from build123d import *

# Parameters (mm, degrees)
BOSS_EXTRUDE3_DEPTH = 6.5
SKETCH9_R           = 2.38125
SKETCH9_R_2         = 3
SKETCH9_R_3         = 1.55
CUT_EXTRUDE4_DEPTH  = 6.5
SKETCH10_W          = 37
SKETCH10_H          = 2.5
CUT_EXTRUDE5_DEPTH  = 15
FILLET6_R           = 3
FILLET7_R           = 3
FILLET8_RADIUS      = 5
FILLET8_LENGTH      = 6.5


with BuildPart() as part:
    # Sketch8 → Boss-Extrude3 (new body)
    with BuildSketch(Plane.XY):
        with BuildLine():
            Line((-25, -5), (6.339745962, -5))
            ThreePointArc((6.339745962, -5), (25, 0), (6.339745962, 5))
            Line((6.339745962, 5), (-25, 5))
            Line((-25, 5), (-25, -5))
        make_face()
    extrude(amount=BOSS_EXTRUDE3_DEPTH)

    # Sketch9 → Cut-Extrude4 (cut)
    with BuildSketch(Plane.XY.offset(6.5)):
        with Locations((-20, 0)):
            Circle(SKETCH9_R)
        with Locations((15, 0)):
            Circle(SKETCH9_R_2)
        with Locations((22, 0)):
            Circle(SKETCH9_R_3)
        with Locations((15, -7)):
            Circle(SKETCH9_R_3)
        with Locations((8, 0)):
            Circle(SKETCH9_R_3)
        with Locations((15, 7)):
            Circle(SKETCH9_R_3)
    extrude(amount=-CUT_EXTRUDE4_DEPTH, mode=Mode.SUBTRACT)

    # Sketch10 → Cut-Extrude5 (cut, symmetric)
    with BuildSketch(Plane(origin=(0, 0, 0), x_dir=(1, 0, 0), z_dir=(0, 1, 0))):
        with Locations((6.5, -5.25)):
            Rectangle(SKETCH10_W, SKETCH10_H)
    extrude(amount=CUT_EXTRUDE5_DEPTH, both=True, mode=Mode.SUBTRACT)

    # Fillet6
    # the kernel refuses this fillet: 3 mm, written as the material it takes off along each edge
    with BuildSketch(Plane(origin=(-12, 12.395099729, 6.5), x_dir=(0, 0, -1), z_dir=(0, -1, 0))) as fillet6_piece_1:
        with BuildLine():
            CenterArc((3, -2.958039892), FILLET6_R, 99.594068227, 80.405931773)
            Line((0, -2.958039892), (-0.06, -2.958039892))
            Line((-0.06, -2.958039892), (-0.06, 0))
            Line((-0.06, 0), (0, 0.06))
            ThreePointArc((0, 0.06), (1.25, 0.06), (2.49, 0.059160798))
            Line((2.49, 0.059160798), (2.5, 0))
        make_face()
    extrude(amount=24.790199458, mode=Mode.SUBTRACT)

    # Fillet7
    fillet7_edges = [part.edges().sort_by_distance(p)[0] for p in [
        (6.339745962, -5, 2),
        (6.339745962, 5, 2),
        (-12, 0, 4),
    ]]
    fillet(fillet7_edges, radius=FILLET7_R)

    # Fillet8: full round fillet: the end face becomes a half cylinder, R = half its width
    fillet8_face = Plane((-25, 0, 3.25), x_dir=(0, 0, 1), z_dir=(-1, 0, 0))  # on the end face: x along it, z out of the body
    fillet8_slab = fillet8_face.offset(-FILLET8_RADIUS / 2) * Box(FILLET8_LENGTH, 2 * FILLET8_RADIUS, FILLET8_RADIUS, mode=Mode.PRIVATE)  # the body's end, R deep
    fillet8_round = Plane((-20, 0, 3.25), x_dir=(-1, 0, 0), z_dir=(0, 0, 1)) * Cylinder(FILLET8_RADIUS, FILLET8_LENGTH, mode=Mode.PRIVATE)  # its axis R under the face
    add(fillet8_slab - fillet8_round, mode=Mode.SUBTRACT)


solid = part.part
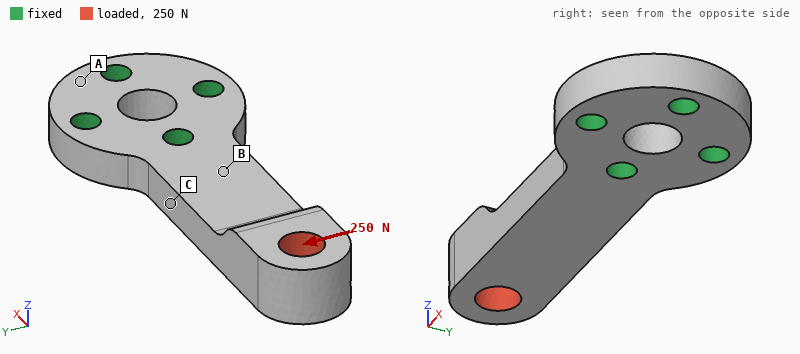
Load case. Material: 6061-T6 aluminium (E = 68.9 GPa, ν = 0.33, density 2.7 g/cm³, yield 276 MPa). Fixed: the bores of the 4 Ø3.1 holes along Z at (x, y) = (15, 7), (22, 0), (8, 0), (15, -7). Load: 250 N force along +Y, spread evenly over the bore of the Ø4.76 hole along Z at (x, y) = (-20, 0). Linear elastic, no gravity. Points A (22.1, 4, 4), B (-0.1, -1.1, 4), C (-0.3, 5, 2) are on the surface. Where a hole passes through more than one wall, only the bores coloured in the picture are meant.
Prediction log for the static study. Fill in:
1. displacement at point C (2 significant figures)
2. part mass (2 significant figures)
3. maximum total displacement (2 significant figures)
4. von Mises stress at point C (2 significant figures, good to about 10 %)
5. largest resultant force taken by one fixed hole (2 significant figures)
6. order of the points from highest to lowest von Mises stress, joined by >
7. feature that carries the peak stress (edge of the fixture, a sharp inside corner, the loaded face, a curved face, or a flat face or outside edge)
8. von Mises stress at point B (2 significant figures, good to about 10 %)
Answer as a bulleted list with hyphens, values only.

- 0.018 mm
- 6.4 g
- 0.12 mm
- 75 MPa
- 410 N
- C > B > A
- a curved face
- 32 MPa
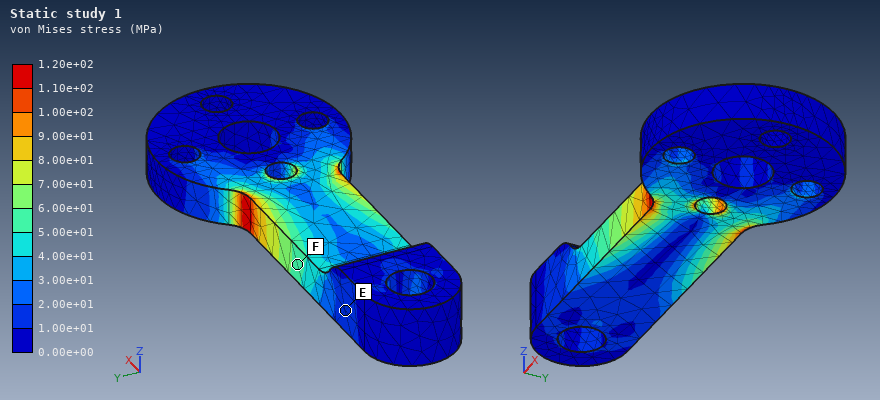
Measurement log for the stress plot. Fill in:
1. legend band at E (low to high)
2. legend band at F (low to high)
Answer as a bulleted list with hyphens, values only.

- 1.00e+01 to 2.00e+01 MPa
- 5.00e+01 to 6.00e+01 MPa
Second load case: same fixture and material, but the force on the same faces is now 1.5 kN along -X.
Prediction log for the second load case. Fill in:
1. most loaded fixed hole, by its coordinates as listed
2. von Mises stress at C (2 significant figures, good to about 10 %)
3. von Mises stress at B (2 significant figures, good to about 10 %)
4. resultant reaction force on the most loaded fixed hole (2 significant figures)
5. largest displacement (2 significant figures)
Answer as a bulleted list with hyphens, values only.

- (8, 0)
- 36 MPa
- 110 MPa
- 1.1 kN
- 0.23 mm
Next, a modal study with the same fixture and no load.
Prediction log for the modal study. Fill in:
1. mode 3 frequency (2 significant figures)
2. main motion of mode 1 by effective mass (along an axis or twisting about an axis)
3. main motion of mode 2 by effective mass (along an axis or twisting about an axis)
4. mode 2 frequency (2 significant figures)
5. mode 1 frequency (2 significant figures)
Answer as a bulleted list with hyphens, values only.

- 14 kHz
- along Z
- along Y
- 6300 Hz
- 2900 Hz
